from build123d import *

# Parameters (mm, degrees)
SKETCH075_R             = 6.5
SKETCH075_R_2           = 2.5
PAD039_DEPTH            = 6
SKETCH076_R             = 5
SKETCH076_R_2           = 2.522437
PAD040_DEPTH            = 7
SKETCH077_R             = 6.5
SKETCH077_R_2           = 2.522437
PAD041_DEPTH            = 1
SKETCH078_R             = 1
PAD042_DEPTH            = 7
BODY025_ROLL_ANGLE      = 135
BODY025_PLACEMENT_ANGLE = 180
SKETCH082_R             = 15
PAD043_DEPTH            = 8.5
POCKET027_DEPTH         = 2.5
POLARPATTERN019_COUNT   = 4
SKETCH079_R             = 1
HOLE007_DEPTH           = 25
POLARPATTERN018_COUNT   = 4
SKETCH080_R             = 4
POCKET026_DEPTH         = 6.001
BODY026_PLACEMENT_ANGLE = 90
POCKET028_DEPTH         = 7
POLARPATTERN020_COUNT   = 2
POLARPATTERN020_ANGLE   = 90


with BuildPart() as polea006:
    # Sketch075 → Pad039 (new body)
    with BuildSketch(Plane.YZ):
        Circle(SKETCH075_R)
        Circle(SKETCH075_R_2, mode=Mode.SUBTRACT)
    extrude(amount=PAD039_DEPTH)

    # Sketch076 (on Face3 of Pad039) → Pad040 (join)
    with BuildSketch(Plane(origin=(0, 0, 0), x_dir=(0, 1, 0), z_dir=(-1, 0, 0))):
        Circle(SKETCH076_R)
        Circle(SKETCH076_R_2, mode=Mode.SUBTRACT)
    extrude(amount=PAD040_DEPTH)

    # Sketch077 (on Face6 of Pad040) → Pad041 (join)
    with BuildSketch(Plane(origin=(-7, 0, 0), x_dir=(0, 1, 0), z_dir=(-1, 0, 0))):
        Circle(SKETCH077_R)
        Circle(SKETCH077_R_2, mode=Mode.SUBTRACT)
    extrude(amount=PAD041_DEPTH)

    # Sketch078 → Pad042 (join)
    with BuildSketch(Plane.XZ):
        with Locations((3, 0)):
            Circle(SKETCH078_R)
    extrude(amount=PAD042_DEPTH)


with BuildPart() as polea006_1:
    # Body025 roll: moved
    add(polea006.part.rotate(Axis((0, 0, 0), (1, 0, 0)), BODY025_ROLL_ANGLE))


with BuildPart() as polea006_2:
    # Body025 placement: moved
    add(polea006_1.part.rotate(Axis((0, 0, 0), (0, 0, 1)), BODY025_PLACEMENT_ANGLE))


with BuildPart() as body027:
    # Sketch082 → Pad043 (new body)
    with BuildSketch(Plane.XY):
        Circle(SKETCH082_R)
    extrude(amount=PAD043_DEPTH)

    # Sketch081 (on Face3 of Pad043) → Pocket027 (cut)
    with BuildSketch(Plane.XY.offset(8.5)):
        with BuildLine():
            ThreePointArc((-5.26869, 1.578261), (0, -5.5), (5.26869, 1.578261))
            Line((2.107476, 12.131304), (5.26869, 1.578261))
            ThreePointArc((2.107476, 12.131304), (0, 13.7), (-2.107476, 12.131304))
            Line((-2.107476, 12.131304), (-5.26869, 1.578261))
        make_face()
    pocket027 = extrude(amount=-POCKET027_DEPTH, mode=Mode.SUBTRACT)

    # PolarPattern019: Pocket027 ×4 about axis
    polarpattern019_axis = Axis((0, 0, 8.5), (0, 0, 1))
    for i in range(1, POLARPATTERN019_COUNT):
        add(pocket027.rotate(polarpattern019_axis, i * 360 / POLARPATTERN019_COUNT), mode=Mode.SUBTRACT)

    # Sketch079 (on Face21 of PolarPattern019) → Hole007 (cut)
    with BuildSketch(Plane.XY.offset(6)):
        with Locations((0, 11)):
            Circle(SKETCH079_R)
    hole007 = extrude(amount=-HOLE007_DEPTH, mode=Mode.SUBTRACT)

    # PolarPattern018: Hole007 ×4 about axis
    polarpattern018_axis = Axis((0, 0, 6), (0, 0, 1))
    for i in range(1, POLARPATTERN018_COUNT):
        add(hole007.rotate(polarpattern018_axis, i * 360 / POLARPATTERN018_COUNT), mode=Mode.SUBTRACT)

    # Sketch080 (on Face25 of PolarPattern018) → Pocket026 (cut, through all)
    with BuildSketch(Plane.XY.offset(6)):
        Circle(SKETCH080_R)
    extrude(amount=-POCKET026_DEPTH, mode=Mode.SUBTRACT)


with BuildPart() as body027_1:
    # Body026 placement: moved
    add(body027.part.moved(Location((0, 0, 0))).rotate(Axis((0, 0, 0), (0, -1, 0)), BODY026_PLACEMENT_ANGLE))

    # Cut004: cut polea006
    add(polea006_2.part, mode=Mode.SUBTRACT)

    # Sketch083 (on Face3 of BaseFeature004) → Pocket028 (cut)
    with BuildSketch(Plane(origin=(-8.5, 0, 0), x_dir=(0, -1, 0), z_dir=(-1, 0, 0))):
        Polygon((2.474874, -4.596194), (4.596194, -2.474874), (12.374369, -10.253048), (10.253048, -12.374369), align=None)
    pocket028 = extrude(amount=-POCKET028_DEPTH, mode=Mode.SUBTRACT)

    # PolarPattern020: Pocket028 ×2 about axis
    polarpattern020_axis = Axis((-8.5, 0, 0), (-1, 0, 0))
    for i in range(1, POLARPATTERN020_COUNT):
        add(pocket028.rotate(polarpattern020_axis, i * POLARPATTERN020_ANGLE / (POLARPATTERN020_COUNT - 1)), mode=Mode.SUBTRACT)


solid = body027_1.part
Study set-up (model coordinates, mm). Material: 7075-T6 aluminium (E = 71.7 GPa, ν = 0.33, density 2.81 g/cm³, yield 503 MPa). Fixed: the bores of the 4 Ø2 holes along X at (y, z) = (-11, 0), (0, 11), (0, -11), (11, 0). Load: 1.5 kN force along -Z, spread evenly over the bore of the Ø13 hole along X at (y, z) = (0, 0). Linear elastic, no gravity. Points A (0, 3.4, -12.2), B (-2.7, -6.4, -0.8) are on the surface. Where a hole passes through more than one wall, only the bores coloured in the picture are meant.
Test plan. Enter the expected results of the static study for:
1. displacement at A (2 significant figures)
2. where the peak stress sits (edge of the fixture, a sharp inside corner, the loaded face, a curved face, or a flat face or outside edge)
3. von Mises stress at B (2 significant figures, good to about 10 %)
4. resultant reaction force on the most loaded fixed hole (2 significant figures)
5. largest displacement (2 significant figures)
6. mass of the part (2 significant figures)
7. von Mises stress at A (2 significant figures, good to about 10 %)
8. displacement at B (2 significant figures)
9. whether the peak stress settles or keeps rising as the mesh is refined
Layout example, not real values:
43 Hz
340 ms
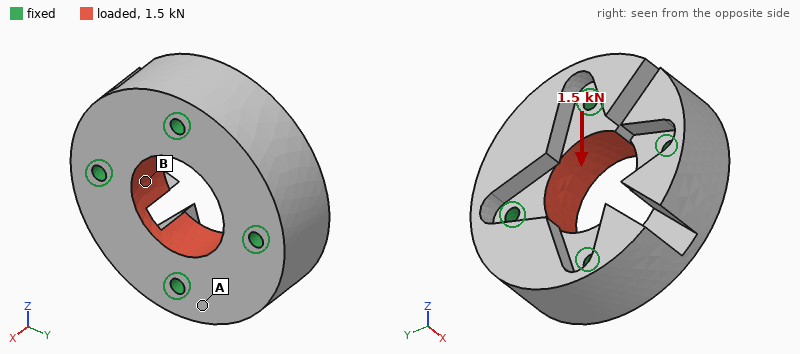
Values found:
0.42 µm
edge of the fixture
12 MPa
410 N
2.0 µm
11 g
5.4 MPa
1.5 µm
keeps rising
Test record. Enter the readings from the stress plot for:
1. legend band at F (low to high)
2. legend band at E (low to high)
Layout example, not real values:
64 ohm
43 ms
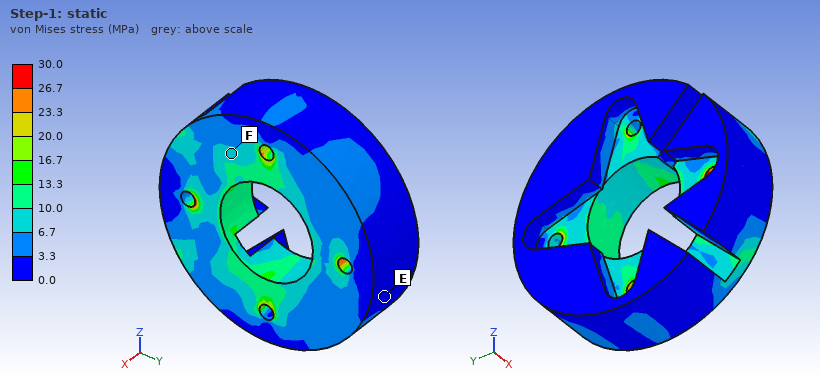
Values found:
6.7 to 10.0 MPa
0.0 to 3.3 MPa
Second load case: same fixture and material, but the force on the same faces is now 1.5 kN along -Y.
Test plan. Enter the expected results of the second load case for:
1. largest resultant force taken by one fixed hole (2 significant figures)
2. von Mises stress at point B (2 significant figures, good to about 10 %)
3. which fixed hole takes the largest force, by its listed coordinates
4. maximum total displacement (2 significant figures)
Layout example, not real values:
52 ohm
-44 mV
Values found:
440 N
10 MPa
(11, 0)
1.8 µm
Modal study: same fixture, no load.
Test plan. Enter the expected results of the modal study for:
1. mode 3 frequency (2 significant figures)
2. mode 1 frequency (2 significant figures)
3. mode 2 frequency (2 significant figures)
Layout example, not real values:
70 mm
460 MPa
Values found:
47 kHz
42 kHz
46 kHz
